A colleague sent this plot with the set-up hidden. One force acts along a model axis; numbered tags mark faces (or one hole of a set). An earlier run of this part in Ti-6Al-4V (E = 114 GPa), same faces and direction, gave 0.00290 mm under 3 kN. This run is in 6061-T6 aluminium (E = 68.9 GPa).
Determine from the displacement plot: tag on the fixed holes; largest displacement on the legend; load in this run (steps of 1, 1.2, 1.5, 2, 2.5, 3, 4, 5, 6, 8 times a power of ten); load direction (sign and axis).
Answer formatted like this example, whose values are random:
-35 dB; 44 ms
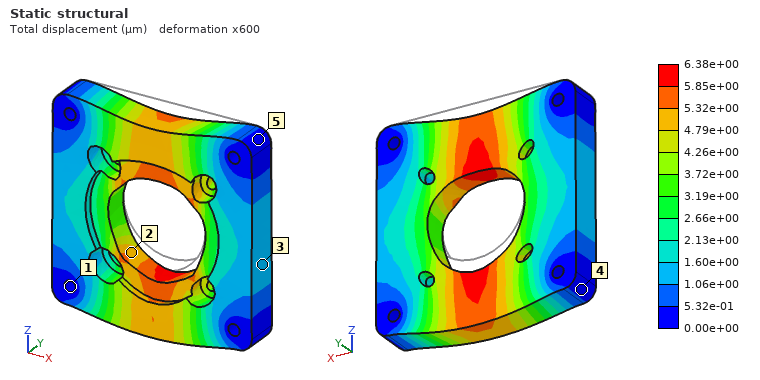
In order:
1; 6.38e+00 µm; 4 kN; -Z
